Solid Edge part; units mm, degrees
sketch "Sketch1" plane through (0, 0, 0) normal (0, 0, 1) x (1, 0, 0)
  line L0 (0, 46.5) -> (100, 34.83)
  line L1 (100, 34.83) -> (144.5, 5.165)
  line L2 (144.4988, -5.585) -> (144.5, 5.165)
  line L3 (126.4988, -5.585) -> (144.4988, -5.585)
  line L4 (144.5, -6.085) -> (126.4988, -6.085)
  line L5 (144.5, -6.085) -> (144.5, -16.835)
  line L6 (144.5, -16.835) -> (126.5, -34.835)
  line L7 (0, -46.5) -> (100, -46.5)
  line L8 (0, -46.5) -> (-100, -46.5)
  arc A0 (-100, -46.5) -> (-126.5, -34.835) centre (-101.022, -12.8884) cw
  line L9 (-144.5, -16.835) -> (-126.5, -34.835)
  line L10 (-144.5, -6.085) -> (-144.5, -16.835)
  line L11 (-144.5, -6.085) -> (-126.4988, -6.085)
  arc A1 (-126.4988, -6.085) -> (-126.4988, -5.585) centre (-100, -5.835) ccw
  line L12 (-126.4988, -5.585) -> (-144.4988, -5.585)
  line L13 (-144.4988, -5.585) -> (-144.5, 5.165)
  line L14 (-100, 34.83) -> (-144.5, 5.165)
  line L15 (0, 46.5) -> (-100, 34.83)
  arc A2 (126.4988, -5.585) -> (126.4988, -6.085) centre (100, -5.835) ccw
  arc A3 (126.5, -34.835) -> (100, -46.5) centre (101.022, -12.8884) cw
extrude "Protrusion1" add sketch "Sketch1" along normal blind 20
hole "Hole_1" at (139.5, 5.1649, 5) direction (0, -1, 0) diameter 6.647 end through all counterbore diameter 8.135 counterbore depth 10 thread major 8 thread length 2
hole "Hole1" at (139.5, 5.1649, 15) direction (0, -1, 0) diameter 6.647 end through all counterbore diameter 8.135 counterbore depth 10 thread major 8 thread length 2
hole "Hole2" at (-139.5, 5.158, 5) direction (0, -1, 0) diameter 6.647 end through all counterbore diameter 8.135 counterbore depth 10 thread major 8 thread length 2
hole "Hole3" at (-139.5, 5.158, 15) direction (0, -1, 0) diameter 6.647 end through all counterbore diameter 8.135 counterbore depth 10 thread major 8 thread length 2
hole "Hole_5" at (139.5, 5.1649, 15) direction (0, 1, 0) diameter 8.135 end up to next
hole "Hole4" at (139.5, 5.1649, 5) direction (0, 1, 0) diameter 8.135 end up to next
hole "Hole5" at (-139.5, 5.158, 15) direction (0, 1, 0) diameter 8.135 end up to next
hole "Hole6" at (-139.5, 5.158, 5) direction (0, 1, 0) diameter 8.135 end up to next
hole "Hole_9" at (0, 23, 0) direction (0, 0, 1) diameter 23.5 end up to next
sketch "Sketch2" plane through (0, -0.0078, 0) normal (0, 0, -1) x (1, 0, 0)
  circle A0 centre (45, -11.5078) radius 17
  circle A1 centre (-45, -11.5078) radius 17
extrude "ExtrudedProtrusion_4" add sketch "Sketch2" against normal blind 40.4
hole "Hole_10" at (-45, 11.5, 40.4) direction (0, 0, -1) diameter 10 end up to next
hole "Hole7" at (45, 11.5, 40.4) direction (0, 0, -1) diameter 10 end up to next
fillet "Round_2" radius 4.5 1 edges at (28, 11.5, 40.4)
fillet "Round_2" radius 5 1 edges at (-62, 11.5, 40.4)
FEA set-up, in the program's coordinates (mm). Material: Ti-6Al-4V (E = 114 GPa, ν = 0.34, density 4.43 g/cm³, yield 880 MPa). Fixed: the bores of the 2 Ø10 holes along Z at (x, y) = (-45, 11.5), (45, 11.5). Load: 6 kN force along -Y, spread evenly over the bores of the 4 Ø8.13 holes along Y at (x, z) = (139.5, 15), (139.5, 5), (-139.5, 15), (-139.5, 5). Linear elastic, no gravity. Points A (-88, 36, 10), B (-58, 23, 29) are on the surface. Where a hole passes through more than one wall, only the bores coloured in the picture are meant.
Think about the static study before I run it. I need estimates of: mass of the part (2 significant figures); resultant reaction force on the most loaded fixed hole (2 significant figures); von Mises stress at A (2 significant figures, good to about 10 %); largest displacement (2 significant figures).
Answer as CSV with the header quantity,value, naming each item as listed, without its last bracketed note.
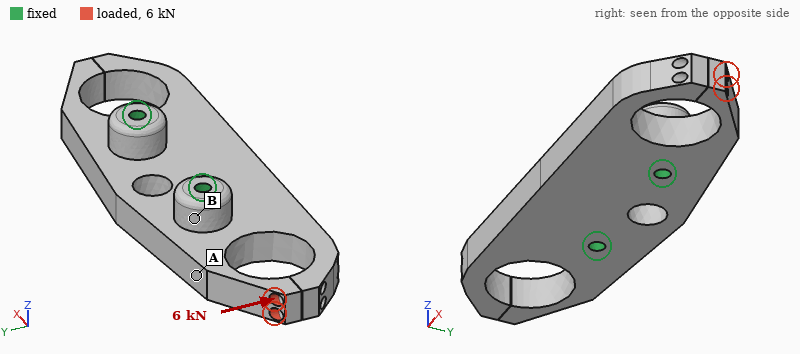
quantity,value
mass of the part,1.7 kg
resultant reaction force on the most loaded fixed hole,3.1 kN
von Mises stress at A,130 MPa
largest displacement,1.0 mm
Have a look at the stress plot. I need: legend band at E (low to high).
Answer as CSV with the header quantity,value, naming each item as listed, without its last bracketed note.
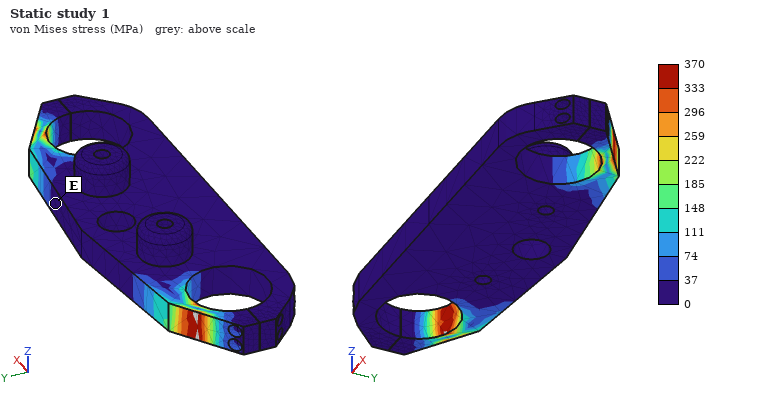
quantity,value
legend band at E,0 to 37 MPa
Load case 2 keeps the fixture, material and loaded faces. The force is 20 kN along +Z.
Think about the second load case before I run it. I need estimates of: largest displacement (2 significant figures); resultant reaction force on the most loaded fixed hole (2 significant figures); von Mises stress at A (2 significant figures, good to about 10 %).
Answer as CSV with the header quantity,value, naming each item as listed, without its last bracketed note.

quantity,value
largest displacement,2.0 mm
resultant reaction force on the most loaded fixed hole,11 kN
von Mises stress at A,140 MPa
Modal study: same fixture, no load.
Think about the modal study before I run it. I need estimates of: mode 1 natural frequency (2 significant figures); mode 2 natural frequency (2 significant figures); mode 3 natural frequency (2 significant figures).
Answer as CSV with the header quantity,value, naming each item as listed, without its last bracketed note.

quantity,value
mode 1 natural frequency,1800 Hz
mode 2 natural frequency,1800 Hz
mode 3 natural frequency,2000 Hz
